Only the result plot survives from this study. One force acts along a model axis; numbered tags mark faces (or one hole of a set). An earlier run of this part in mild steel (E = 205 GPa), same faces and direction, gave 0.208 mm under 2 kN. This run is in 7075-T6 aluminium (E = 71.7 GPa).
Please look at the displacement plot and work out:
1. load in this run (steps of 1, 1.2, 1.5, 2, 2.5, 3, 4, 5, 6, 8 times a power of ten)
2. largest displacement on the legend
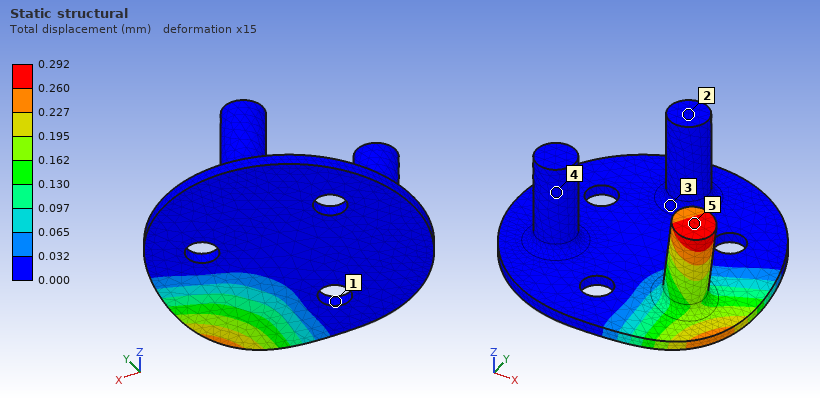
1 kN
0.292 mm
